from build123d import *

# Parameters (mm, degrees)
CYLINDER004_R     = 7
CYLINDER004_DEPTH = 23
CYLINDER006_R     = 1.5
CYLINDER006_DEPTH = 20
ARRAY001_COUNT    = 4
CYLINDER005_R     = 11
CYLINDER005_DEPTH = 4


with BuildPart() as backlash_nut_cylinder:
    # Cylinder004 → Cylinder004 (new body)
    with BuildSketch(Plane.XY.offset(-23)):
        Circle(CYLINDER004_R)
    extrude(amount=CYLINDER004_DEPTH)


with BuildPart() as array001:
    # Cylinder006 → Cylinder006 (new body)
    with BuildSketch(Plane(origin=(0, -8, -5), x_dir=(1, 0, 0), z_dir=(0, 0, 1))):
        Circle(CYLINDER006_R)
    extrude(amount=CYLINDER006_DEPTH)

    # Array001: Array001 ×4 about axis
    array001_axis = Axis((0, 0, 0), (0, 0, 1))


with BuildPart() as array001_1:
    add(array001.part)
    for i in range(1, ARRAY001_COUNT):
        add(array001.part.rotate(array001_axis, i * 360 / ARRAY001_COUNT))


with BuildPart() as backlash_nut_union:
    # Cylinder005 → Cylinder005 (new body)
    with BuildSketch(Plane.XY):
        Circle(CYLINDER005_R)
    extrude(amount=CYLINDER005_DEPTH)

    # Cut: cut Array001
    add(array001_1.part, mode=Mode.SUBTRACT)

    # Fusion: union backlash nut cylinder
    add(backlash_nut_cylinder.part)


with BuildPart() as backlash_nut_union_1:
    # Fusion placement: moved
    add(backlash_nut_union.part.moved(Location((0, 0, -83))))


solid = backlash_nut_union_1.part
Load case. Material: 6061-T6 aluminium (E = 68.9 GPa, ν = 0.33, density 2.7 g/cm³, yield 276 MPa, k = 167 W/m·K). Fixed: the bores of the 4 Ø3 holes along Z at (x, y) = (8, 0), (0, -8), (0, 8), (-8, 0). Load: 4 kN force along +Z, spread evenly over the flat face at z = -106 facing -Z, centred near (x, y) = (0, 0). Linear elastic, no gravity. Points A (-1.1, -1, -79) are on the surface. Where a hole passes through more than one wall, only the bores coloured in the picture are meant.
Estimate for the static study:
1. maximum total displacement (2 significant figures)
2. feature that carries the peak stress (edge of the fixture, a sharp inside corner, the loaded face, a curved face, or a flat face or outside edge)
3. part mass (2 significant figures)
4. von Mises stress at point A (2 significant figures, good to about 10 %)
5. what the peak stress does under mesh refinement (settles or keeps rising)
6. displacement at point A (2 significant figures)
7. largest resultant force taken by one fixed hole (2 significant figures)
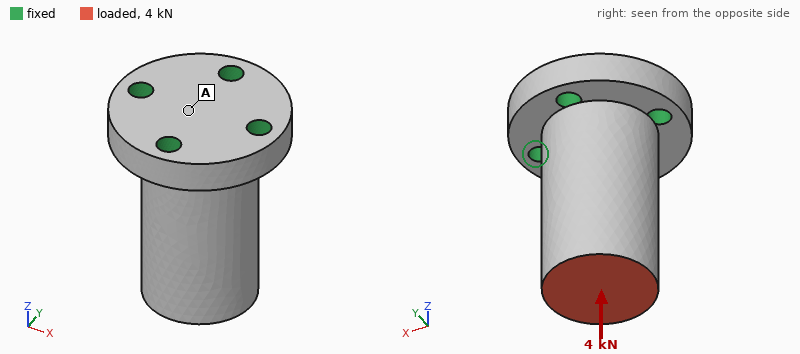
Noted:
11 µm
edge of the fixture
13 g
16 MPa
keeps rising
3.2 µm
1.0 kN
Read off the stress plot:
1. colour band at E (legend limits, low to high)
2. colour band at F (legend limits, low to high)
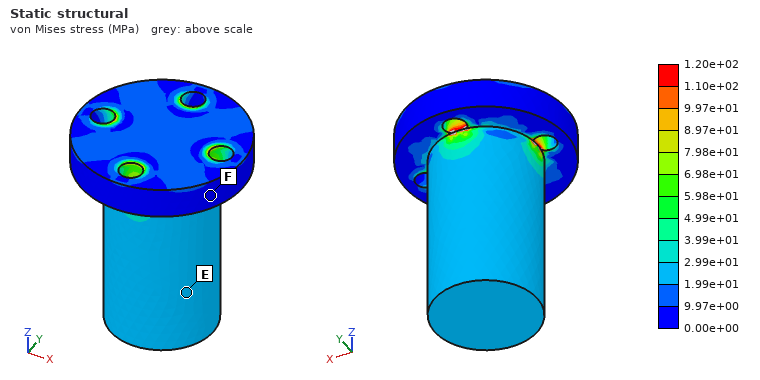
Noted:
1.99e+01 to 2.99e+01 MPa
0.00e+00 to 9.97e+00 MPa
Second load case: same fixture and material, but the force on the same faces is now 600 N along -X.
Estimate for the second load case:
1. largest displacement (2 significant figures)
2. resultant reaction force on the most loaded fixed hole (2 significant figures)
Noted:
32 µm
990 N
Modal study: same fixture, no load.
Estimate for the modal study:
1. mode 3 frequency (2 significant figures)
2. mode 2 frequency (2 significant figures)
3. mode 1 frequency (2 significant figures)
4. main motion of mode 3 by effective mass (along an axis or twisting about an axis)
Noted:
32 kHz
13 kHz
13 kHz
twisting about Z
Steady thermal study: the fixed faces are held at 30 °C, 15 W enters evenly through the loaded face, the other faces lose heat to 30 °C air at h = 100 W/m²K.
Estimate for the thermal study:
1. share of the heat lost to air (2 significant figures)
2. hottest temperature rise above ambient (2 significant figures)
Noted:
5.7 %
15 K
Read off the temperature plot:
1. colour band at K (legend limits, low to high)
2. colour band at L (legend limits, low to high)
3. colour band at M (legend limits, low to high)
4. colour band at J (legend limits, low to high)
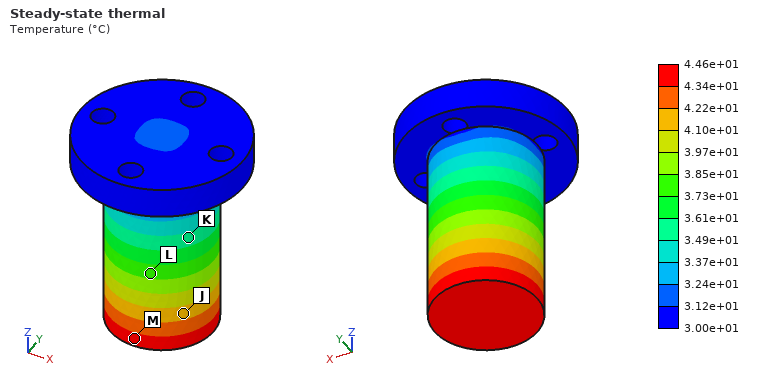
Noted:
3.49e+01 to 3.61e+01 °C
3.73e+01 to 3.85e+01 °C
4.34e+01 to 4.46e+01 °C
4.10e+01 to 4.22e+01 °C
